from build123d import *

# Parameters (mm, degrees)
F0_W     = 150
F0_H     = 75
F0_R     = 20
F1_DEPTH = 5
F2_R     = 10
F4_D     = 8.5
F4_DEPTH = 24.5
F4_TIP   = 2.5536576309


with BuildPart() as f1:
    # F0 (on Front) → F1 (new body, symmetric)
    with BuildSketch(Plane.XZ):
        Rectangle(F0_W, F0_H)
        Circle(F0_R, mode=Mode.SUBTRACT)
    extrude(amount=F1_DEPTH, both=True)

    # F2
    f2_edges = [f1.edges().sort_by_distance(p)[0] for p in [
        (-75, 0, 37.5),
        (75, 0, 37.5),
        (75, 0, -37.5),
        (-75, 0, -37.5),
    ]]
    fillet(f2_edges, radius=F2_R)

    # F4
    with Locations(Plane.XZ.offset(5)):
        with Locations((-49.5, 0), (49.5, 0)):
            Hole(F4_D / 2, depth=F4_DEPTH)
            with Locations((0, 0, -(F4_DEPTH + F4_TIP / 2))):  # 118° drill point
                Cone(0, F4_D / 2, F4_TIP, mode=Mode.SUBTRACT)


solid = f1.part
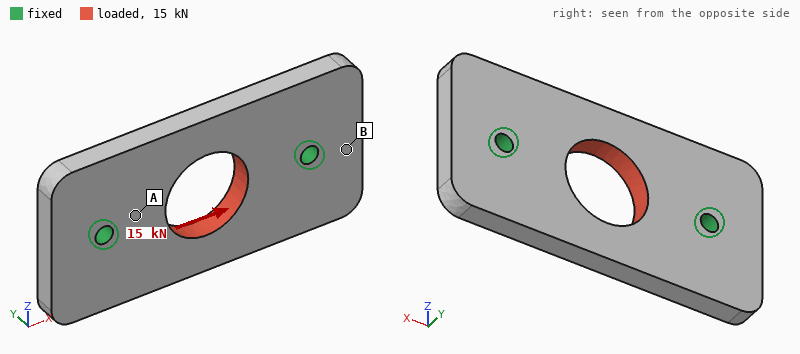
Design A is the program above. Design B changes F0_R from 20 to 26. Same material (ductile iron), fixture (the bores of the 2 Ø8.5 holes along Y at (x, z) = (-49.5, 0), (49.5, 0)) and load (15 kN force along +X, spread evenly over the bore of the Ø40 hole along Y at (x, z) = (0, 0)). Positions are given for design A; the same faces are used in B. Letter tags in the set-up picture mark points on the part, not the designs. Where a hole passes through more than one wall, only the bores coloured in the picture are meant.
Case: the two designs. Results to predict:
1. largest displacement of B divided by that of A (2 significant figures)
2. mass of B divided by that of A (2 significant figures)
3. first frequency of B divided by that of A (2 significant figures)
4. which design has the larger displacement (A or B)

1.2
0.91
1.0
B
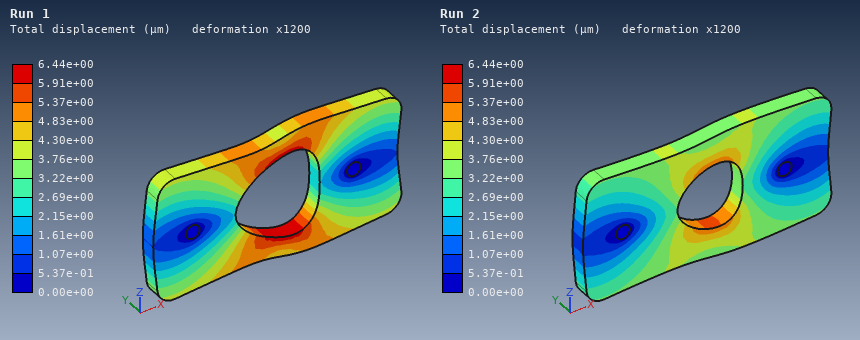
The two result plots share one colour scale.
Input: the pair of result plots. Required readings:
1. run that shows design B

Run 1
